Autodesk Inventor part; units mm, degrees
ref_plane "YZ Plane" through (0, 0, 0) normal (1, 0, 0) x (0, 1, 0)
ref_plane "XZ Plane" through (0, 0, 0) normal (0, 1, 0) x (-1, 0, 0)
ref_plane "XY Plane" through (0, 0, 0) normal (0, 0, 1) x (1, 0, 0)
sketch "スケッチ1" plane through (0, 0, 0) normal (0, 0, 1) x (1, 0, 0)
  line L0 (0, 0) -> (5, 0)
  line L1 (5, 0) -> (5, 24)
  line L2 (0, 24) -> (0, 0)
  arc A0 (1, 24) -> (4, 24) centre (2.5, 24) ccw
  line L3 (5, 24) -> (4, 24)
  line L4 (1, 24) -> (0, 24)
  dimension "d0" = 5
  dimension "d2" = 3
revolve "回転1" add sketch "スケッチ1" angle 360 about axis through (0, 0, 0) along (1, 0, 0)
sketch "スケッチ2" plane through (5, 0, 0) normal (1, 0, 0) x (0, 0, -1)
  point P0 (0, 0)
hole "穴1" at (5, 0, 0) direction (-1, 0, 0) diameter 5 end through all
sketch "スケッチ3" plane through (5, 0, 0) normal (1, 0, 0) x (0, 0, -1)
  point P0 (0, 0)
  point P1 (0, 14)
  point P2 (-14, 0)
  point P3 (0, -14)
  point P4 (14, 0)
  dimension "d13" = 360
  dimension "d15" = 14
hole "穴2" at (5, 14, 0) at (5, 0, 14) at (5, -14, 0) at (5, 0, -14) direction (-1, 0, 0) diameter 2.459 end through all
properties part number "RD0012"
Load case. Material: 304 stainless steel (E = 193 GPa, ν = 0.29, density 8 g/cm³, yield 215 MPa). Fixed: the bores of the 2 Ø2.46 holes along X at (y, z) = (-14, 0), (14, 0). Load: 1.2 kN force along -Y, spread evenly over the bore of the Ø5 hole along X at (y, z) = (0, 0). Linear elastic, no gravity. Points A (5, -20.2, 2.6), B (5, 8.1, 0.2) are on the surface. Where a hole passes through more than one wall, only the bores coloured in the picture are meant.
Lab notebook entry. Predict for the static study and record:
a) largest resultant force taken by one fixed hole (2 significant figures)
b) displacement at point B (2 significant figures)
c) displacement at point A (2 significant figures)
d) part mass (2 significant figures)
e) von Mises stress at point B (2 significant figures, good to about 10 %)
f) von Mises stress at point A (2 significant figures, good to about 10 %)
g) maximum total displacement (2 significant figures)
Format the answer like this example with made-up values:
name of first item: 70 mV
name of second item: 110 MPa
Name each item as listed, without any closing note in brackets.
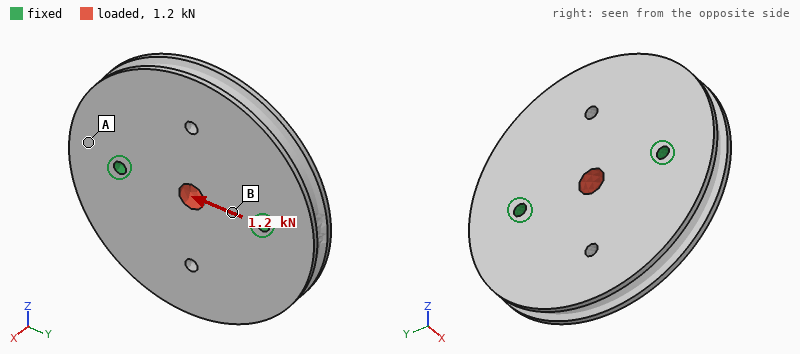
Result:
largest resultant force taken by one fixed hole: 600 N
displacement at point B: 0.39 µm
displacement at point A: 0.15 µm
part mass: 67 g
von Mises stress at point B: 13 MPa
von Mises stress at point A: 2.6 MPa
maximum total displacement: 0.85 µm
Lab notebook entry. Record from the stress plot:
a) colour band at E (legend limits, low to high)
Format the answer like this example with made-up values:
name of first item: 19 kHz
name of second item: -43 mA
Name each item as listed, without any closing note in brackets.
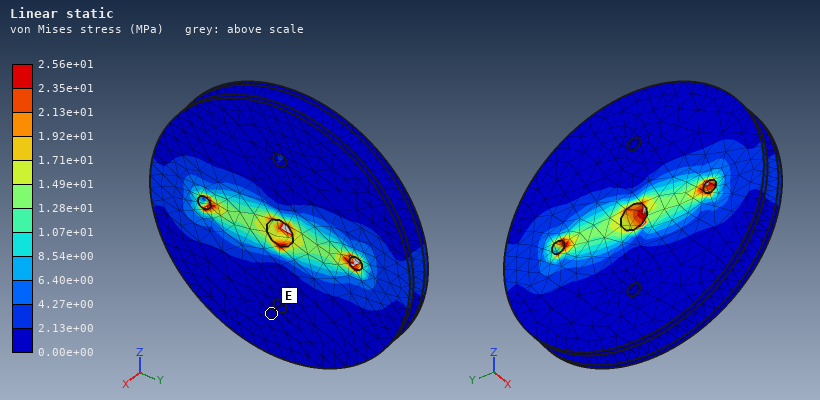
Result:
colour band at E: 0.00e+00 to 2.13e+00 MPa
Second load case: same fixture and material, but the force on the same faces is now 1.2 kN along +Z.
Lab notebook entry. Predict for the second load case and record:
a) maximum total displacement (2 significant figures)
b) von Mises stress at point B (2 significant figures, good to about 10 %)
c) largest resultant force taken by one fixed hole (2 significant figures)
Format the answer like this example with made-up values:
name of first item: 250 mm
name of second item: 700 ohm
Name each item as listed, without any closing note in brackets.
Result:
maximum total displacement: 1.1 µm
von Mises stress at point B: 5.8 MPa
largest resultant force taken by one fixed hole: 600 N
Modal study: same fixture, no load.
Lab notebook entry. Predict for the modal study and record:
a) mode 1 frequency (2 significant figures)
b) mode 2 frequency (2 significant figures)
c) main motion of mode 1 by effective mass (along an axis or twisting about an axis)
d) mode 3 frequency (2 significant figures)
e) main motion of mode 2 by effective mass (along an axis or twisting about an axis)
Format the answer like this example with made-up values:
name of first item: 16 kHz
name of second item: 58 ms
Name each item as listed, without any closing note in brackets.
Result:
mode 1 frequency: 6300 Hz
mode 2 frequency: 8600 Hz
main motion of mode 1 by effective mass: twisting about Y
mode 3 frequency: 15 kHz
main motion of mode 2 by effective mass: along X
